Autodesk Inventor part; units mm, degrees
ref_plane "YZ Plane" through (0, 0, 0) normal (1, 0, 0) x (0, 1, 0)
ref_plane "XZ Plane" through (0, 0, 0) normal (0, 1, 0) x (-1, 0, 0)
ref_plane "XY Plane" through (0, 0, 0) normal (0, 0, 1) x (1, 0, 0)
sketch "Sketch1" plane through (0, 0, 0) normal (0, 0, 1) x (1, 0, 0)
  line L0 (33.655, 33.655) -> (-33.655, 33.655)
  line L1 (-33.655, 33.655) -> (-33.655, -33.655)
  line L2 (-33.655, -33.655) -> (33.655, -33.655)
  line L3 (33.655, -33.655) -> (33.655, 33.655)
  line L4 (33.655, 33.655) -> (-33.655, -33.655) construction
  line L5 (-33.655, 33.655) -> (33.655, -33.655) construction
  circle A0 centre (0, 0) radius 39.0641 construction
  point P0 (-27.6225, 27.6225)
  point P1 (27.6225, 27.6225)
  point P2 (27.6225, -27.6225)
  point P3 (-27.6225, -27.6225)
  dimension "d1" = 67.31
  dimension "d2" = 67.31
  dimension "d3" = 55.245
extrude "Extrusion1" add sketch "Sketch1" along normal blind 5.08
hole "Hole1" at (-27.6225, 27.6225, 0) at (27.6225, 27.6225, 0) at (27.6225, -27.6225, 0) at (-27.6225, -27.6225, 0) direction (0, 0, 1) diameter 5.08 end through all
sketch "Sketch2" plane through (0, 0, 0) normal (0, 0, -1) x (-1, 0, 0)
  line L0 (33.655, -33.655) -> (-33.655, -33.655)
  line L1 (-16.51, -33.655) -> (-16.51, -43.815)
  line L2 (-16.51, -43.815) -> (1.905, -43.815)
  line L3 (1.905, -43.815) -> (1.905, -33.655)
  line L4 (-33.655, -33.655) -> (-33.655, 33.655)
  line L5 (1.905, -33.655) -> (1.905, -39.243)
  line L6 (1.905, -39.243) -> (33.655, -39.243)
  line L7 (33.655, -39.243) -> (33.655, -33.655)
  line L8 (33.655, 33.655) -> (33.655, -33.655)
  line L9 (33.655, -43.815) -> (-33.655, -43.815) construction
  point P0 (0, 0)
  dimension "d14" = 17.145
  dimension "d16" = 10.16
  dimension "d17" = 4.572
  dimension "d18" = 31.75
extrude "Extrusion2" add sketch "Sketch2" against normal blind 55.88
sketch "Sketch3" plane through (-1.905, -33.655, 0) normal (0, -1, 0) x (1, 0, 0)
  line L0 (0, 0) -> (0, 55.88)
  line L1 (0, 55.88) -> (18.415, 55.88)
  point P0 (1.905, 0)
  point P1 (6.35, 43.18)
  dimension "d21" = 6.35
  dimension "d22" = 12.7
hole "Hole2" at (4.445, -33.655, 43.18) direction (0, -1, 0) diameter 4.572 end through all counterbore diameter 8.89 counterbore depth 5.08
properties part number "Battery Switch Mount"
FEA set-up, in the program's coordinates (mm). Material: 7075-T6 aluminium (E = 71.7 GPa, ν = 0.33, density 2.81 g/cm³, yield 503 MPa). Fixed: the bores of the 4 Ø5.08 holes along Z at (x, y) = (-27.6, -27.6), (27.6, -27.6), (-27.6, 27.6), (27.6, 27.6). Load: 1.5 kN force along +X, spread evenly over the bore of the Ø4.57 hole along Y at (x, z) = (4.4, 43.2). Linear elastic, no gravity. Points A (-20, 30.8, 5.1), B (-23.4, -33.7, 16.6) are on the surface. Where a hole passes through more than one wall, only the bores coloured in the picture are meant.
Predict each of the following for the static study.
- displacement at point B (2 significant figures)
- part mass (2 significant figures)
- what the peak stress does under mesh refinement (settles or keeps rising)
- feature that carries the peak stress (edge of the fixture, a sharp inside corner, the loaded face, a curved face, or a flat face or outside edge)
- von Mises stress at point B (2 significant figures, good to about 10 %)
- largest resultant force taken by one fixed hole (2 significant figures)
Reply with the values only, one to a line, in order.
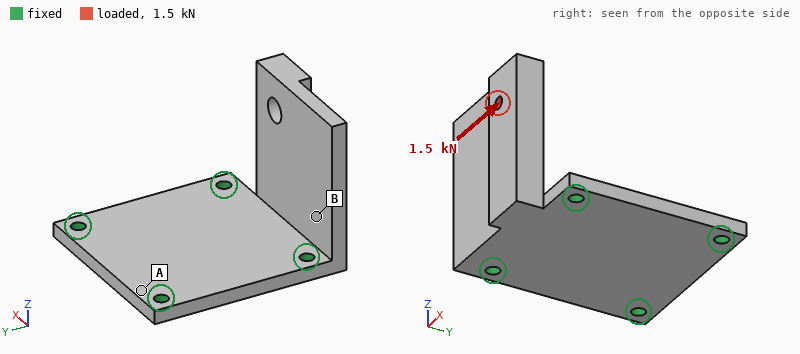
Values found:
0.034 mm
120 g
keeps rising
a sharp inside corner
26 MPa
1.5 kN
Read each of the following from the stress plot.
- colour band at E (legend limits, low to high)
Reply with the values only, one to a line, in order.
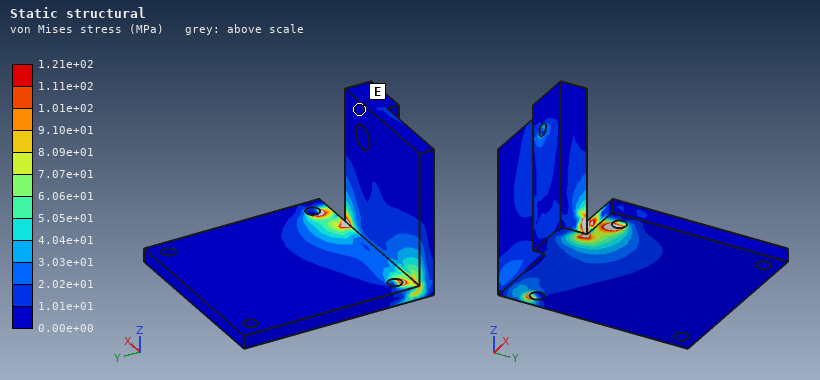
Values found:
0.00e+00 to 1.01e+01 MPa
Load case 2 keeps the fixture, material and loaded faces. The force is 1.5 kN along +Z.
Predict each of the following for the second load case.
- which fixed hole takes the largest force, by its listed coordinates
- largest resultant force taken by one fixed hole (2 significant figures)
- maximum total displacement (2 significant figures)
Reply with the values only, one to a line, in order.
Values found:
(27.6, -27.6)
1.0 kN
0.39 mm
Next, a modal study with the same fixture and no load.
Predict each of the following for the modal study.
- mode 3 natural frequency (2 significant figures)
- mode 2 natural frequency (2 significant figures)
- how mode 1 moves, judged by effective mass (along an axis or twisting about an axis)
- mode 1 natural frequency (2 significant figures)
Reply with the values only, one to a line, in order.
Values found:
4300 Hz
3100 Hz
along Y
1100 Hz
